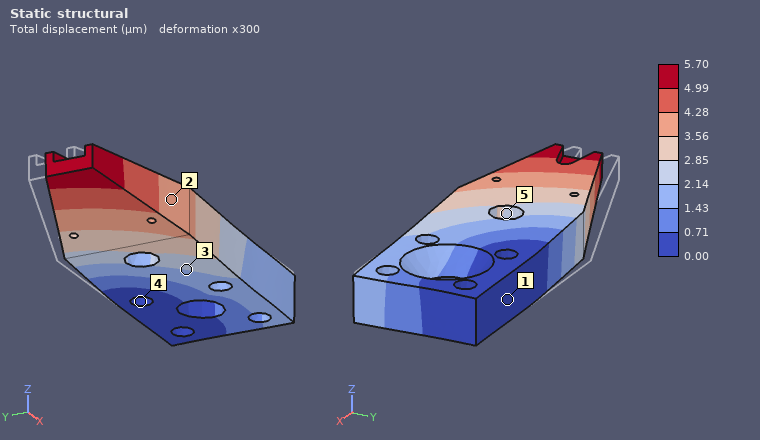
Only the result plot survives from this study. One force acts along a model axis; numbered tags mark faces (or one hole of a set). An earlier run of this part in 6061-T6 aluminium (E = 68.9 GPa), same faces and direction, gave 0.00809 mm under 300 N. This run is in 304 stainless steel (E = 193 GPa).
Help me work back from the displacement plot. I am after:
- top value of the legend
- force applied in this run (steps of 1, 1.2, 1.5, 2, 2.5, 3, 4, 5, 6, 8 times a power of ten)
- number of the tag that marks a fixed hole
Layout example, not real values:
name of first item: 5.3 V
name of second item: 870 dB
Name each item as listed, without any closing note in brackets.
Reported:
top value of the legend: 5.70 µm
force applied in this run: 600 N
number of the tag that marks a fixed hole: 4
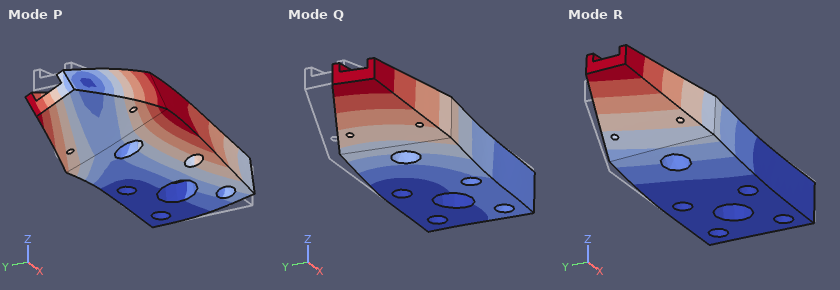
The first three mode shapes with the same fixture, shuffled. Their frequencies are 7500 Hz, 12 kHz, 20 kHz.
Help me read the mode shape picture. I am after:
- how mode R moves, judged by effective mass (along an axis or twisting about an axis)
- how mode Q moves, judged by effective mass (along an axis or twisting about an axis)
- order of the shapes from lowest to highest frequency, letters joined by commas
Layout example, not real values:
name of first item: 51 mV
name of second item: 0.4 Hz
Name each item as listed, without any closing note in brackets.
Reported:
how mode R moves, judged by effective mass: along Z
how mode Q moves, judged by effective mass: along Y
order of the shapes from lowest to highest frequency, letters joined by commas: R, Q, P
